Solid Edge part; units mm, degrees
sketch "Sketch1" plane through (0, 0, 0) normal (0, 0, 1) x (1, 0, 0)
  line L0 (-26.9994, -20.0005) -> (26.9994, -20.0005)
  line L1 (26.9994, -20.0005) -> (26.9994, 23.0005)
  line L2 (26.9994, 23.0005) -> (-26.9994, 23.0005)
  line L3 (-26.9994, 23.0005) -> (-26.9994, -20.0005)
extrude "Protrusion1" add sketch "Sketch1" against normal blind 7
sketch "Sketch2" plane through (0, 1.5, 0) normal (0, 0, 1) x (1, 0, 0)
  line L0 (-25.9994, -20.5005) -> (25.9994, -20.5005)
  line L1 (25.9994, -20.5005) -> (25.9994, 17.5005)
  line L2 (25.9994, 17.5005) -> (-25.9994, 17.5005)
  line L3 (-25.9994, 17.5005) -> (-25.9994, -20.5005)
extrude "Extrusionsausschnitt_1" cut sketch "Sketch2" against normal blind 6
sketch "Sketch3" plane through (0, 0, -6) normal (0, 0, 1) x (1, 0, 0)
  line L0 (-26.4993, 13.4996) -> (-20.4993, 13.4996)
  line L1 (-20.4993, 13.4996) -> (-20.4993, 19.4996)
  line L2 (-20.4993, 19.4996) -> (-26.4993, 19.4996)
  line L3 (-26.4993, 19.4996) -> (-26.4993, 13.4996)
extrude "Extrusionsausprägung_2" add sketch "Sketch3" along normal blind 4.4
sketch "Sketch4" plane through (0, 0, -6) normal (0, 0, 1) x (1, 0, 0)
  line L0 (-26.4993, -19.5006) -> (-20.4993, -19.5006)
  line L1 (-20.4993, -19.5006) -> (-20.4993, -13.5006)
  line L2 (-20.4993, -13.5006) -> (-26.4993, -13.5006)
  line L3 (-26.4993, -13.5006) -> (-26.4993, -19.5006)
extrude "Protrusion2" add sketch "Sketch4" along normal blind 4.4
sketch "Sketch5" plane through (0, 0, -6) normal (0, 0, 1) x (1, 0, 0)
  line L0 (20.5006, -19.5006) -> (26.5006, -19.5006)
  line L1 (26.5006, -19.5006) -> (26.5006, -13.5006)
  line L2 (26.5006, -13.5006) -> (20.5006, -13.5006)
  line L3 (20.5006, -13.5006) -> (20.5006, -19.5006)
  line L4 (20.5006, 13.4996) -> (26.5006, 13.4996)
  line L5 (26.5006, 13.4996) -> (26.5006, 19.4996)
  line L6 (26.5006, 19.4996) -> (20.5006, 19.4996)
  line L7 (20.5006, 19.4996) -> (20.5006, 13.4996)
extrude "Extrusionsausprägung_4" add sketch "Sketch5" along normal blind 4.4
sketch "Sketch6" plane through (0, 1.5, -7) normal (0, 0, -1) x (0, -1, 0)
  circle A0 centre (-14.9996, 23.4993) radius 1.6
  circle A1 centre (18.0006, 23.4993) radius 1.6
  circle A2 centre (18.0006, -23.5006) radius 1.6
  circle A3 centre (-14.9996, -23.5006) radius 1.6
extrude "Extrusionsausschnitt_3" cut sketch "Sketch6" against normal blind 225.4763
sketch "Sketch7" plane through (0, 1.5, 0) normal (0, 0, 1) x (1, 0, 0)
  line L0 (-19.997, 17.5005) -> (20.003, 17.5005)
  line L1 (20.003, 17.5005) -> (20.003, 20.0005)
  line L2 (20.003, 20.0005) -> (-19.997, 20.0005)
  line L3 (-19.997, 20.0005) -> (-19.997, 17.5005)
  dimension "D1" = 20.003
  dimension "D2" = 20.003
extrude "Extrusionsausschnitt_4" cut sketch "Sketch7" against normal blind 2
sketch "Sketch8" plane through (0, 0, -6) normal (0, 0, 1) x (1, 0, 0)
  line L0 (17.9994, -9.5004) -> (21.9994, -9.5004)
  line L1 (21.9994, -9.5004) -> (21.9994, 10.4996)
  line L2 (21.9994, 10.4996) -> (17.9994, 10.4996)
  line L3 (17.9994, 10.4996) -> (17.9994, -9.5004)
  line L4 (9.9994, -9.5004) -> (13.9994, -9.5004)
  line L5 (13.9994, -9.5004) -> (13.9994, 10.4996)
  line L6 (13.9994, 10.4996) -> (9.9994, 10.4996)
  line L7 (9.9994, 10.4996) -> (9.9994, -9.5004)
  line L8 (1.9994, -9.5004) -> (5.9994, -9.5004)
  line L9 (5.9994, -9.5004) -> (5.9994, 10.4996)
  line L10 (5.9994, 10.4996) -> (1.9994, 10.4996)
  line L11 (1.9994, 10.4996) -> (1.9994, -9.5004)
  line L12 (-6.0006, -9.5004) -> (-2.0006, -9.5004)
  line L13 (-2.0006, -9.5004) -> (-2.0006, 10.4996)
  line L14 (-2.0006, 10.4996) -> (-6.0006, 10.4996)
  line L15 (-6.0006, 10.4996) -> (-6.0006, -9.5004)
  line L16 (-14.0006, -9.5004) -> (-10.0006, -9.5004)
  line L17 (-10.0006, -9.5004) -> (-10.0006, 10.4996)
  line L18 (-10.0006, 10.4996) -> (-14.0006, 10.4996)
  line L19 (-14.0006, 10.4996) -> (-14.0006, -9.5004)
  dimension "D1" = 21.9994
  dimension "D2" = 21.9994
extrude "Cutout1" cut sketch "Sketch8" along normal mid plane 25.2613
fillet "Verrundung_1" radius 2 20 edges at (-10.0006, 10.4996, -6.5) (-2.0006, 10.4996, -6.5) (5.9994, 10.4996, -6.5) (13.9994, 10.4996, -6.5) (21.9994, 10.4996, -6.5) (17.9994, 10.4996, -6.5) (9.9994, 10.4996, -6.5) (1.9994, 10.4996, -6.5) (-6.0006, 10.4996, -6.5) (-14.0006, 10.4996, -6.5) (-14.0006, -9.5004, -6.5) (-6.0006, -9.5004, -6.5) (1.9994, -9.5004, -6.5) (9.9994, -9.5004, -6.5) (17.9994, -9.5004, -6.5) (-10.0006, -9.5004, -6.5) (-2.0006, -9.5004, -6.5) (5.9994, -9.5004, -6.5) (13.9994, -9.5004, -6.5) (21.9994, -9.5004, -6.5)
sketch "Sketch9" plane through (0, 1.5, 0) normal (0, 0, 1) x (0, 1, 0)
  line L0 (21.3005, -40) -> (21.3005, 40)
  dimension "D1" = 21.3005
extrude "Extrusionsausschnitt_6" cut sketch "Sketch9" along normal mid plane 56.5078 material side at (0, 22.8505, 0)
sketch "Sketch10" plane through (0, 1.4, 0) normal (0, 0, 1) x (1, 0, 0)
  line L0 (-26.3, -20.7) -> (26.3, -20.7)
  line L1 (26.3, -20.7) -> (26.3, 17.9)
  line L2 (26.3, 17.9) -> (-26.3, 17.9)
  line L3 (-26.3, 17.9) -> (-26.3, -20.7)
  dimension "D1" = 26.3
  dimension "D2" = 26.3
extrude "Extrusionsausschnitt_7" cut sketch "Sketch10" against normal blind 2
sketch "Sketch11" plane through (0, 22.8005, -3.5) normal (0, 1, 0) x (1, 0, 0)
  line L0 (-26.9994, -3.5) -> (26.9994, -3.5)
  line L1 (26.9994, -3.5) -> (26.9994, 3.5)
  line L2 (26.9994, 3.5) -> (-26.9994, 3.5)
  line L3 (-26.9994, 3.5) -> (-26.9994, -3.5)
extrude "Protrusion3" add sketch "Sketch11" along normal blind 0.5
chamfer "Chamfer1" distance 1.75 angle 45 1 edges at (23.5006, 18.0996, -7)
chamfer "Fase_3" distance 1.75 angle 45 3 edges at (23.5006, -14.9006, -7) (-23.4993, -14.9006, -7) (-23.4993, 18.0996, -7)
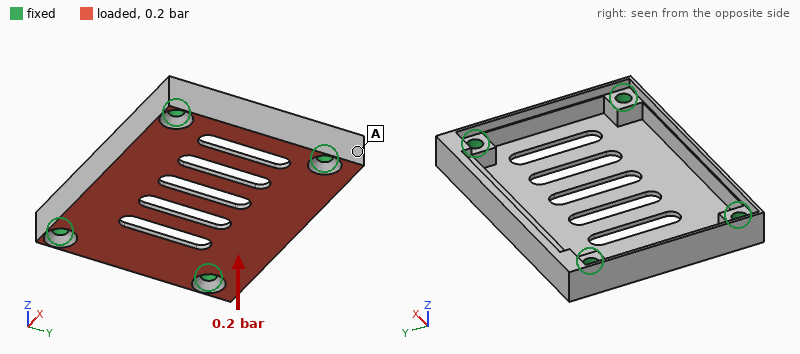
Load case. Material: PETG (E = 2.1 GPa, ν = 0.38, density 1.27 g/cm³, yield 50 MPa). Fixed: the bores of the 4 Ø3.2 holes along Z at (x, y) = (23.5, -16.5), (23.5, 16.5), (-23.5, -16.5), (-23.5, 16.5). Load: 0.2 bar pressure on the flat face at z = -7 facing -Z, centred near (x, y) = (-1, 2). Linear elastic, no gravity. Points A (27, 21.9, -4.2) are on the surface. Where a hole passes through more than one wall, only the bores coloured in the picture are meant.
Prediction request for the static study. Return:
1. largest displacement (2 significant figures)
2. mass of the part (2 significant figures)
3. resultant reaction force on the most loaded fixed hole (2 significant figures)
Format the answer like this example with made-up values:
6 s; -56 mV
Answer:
0.78 mm; 5.2 g; 12 N
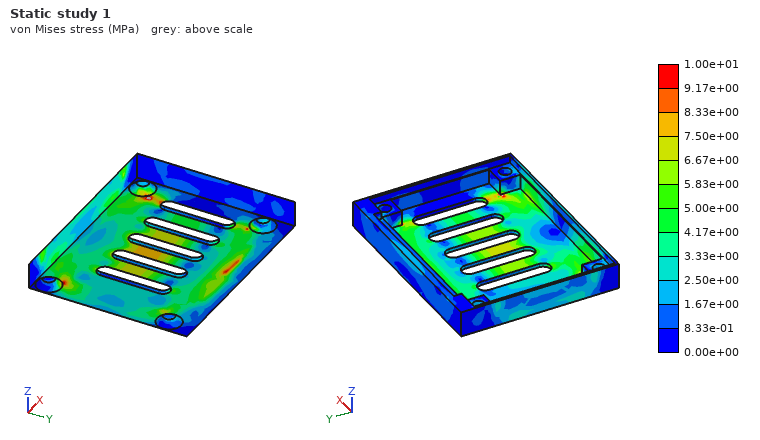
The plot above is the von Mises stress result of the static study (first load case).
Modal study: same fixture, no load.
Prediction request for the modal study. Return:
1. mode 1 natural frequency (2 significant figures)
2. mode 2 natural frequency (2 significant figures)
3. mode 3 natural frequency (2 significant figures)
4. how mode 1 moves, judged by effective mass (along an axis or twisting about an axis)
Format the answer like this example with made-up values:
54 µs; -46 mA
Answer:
940 Hz; 1500 Hz; 1900 Hz; along Z
